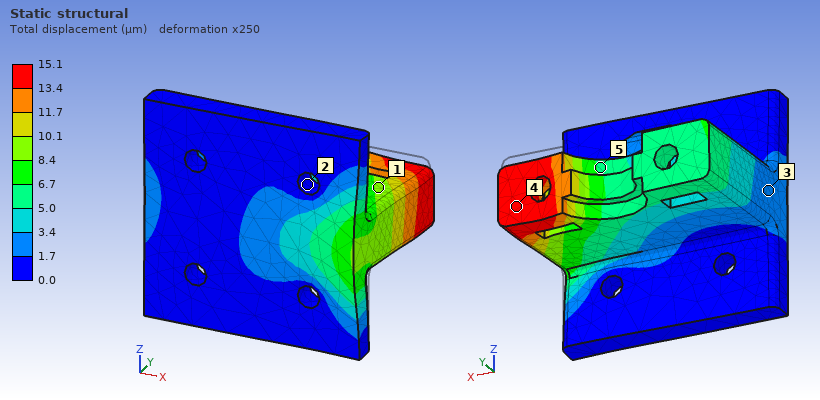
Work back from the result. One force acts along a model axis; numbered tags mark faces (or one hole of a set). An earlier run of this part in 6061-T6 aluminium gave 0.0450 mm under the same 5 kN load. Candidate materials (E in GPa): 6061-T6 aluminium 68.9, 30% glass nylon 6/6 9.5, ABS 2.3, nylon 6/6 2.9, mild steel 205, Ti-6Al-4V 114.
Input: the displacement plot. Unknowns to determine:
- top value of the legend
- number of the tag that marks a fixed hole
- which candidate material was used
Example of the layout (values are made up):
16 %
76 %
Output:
15.1 µm
2
mild steel
